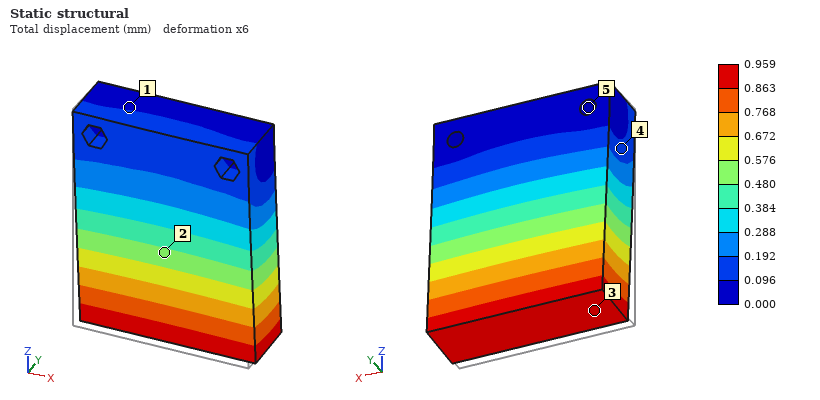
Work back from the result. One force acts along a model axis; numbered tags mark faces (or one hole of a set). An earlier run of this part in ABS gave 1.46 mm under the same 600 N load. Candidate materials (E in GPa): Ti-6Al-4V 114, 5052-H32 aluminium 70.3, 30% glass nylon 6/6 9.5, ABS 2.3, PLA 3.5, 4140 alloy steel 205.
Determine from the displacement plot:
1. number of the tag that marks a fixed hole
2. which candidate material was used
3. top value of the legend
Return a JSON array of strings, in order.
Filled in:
["5", "PLA", "0.959 mm"]
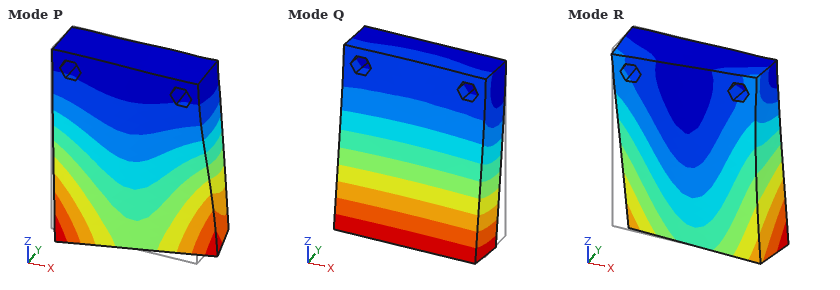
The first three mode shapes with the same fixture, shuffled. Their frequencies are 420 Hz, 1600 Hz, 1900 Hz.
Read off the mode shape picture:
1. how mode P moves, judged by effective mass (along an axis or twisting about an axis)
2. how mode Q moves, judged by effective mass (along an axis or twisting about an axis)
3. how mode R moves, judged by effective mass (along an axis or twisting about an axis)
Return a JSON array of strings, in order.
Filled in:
["along X", "along Y", "along X"]
